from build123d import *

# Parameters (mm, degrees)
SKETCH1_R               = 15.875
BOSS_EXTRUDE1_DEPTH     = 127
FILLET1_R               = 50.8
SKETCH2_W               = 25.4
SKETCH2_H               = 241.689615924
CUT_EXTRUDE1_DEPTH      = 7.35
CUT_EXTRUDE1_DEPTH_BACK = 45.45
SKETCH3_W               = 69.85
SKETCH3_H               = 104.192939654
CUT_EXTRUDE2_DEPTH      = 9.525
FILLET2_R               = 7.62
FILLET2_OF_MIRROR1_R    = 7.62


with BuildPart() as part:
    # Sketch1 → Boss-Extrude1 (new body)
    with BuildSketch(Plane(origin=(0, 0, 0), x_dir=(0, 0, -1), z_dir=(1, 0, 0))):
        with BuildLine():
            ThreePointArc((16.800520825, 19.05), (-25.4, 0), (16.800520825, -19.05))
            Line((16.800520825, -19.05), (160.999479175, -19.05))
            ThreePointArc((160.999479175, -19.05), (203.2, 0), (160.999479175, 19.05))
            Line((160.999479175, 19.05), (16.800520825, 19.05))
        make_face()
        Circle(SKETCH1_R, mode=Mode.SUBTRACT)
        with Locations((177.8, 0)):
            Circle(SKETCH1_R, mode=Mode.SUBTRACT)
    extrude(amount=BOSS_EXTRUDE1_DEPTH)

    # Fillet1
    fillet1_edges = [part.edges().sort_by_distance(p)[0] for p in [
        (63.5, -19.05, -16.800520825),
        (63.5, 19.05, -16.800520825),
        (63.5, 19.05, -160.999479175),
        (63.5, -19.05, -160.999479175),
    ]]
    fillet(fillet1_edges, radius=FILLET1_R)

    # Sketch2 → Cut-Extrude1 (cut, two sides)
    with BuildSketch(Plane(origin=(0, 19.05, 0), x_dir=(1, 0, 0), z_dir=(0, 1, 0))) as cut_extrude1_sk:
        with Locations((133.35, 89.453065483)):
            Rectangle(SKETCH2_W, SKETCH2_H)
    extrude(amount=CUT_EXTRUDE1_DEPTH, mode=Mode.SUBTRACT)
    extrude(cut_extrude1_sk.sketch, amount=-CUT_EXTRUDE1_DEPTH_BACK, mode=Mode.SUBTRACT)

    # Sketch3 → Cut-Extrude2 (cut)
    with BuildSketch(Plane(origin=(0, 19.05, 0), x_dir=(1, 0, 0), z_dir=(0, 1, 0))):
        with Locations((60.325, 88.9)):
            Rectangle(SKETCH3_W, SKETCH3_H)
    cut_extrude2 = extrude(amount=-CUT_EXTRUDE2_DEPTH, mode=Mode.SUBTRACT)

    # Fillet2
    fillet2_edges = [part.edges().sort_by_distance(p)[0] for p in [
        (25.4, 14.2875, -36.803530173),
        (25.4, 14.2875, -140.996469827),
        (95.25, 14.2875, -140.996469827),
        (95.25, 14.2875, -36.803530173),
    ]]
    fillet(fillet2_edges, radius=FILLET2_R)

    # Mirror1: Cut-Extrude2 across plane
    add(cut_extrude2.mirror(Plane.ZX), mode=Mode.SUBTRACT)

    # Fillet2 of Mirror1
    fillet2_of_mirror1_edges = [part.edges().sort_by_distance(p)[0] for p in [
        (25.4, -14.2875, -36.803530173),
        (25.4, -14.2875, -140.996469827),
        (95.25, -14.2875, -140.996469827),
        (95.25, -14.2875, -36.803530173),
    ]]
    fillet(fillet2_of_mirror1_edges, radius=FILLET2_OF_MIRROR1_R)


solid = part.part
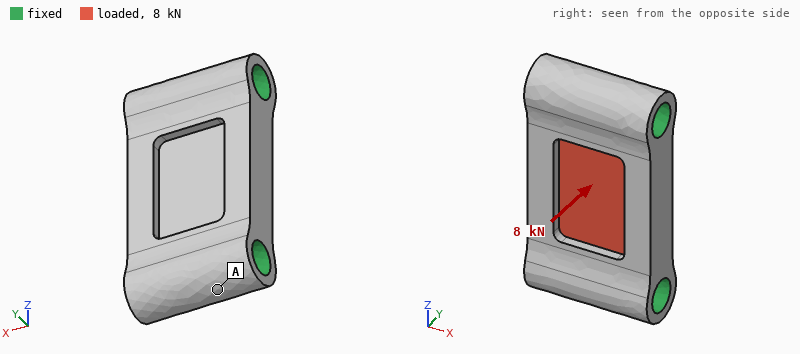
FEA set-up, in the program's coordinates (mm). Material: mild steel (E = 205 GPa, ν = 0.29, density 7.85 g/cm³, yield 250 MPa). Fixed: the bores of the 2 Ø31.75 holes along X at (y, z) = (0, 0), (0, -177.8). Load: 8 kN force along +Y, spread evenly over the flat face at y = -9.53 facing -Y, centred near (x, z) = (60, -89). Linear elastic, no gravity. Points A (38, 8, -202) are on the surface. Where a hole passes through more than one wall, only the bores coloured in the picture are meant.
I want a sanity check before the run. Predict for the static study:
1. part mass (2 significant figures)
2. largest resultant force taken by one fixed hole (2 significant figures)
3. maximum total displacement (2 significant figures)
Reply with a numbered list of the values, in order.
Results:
1. 6.1 kg
2. 4.0 kN
3. 3.4 µm
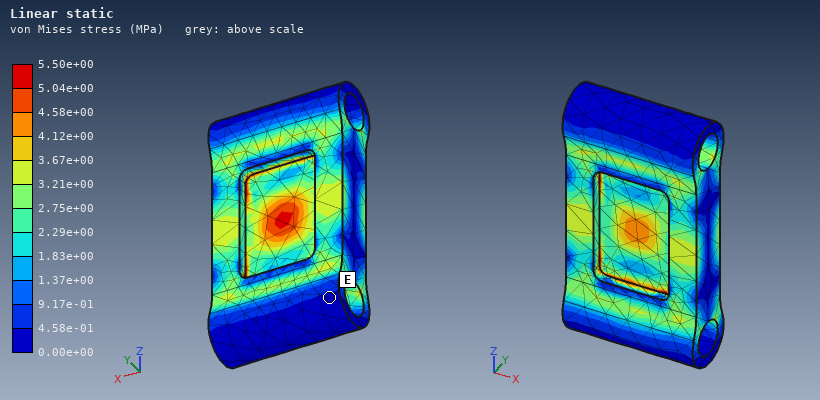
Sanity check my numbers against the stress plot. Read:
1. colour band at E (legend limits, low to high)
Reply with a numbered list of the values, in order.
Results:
1. 0.00e+00 to 4.58e-01 MPa
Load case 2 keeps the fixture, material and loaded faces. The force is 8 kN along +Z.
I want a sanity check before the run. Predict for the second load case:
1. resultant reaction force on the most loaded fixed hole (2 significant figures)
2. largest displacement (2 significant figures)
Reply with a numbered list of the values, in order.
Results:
1. 4.0 kN
2. 0.57 µm
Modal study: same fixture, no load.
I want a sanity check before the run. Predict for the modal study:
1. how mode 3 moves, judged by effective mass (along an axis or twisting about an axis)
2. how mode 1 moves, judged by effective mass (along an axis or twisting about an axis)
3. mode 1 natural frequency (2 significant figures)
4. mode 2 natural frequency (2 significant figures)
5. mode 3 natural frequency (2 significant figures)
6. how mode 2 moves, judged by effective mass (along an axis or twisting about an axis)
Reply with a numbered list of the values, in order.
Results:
1. along X
2. along Y
3. 6400 Hz
4. 7200 Hz
5. 9500 Hz
6. twisting about Z
